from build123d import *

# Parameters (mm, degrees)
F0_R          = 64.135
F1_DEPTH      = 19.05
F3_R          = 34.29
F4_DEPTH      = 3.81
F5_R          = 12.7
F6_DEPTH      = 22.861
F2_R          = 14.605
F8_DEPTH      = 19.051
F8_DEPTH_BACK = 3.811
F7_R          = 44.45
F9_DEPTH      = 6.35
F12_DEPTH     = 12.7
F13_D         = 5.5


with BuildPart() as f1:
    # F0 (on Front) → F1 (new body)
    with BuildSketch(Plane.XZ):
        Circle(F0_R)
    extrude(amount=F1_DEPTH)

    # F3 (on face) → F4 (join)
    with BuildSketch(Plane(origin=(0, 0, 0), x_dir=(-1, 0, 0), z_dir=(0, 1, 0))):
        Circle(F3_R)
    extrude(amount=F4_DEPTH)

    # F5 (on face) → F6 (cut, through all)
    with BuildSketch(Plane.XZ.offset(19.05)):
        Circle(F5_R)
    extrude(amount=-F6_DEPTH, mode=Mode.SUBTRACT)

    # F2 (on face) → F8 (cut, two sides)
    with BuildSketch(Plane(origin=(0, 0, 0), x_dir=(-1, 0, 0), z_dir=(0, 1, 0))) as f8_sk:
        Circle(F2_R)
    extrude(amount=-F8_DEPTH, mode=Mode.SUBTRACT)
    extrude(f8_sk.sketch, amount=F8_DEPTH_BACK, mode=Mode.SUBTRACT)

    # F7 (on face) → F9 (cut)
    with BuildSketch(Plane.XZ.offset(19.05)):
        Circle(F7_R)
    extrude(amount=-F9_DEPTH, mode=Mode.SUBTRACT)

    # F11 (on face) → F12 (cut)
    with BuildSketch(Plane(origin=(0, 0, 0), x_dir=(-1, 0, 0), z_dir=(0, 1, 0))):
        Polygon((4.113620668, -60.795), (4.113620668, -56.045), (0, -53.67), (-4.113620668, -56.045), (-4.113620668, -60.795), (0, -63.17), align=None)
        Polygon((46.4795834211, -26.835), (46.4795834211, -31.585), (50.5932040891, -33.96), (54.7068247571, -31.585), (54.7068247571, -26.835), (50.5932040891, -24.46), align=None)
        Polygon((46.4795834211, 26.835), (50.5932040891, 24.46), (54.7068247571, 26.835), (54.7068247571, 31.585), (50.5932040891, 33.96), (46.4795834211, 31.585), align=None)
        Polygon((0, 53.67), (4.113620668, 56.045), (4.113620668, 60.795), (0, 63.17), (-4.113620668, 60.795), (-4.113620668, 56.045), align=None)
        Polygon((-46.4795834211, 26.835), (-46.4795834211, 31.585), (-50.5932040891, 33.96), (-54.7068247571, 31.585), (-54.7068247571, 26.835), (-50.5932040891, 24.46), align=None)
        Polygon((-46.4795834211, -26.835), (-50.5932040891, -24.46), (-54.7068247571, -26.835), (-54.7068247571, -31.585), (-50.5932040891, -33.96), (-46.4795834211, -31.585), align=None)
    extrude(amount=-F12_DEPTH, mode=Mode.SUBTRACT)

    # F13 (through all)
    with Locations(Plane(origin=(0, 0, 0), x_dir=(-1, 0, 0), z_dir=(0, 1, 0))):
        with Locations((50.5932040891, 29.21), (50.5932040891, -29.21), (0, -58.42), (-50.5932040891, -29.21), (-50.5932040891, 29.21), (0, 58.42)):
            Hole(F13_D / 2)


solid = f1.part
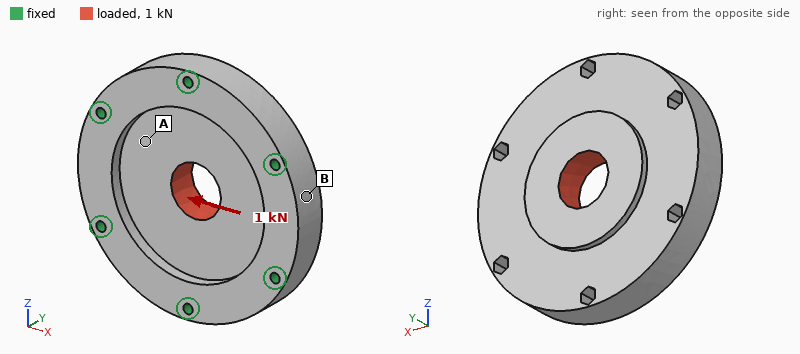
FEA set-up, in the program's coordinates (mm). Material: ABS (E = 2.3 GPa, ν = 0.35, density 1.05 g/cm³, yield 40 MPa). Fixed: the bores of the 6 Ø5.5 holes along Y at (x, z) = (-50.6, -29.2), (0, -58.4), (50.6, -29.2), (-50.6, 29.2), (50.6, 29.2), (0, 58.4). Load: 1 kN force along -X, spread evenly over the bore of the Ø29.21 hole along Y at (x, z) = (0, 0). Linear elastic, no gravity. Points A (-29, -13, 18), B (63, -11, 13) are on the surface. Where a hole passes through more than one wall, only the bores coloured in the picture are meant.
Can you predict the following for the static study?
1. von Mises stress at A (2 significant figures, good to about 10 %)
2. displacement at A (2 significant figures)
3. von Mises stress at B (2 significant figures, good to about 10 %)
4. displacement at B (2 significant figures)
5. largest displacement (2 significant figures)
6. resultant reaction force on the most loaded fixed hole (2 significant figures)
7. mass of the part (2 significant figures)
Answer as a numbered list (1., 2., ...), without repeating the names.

1. 0.82 MPa
2. 15 µm
3. 0.38 MPa
4. 12 µm
5. 24 µm
6. 190 N
7. 210 g
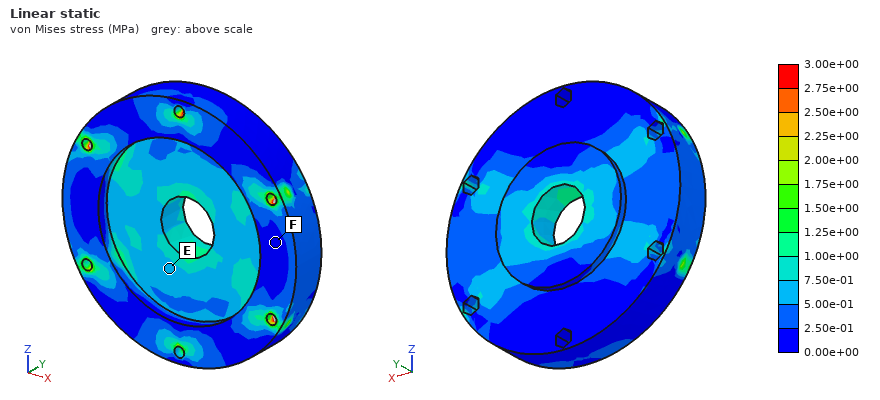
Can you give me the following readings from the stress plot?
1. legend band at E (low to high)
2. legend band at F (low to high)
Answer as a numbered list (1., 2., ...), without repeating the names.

1. 5.00e-01 to 7.50e-01 MPa
2. 0.00e+00 to 2.50e-01 MPa
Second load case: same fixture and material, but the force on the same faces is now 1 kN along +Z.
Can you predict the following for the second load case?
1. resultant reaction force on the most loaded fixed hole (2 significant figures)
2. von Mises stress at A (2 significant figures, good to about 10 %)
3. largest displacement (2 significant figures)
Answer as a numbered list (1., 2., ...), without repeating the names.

1. 200 N
2. 0.62 MPa
3. 23 µm
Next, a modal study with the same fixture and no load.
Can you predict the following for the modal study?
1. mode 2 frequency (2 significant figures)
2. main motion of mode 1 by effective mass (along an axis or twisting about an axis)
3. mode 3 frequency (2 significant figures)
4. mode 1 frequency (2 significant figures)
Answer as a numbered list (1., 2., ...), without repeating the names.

1. 3200 Hz
2. along Y
3. 3200 Hz
4. 2200 Hz
